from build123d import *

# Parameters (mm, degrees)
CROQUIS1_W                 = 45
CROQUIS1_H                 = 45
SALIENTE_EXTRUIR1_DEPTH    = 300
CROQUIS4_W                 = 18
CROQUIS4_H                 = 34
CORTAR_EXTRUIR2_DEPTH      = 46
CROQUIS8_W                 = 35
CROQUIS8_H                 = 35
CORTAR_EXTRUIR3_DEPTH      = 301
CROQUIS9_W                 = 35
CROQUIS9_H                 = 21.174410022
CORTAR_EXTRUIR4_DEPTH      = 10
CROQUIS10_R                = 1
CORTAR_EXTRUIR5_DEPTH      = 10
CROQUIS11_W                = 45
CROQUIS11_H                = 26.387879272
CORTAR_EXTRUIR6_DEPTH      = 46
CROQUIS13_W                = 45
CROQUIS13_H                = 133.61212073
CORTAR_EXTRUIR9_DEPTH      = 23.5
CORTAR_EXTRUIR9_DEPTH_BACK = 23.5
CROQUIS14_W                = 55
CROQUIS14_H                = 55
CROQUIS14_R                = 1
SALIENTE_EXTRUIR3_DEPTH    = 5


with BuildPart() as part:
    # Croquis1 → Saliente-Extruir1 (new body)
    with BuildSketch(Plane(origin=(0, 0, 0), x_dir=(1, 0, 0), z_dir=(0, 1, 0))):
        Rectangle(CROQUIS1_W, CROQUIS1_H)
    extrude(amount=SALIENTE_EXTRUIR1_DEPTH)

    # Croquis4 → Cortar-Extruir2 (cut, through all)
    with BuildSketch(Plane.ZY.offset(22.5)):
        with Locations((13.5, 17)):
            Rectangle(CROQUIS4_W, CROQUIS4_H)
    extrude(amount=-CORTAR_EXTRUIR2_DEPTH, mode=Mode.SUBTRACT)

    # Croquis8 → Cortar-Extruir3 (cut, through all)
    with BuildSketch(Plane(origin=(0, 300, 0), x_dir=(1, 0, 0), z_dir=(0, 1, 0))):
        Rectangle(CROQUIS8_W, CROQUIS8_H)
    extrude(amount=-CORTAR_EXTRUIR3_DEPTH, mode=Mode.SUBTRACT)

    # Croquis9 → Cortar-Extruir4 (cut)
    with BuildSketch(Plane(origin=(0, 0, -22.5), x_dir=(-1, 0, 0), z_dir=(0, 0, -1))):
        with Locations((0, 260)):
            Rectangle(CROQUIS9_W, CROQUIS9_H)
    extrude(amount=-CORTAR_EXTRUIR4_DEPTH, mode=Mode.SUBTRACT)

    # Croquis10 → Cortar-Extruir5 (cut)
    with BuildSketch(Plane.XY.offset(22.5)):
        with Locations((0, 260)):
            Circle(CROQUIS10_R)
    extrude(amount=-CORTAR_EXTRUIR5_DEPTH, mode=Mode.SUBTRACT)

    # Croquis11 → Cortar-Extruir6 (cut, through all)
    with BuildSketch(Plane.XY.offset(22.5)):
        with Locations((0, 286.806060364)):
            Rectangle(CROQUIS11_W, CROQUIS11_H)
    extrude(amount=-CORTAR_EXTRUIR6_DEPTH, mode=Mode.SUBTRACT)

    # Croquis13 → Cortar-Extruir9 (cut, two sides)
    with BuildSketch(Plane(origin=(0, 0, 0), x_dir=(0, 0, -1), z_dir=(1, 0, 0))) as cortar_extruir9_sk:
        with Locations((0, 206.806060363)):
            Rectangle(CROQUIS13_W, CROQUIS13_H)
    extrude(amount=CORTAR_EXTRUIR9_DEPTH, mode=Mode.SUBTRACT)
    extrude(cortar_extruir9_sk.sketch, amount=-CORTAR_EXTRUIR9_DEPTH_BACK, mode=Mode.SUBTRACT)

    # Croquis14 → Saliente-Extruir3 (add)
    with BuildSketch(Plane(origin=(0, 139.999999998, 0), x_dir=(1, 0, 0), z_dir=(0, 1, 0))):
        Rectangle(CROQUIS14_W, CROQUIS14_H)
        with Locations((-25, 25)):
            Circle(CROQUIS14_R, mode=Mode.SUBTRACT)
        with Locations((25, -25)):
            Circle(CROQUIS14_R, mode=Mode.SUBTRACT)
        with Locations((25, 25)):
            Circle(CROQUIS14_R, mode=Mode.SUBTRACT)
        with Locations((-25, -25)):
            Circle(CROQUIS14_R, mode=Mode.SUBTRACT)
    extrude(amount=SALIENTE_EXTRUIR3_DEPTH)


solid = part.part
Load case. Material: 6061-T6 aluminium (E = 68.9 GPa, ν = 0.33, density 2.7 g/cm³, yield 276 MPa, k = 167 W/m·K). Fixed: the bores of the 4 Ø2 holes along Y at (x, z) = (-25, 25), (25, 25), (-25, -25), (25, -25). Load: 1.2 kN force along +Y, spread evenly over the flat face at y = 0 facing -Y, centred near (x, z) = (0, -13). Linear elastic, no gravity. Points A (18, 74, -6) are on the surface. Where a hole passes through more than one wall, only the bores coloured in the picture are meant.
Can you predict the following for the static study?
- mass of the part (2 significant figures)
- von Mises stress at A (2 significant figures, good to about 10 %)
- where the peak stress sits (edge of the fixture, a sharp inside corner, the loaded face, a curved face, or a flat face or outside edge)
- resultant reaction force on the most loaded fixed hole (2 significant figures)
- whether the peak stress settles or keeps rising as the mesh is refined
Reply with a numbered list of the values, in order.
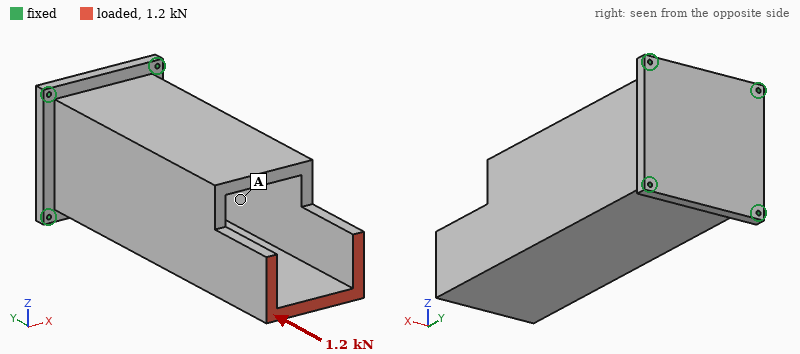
1. 310 g
2. 2.0 MPa
3. edge of the fixture
4. 490 N
5. keeps rising
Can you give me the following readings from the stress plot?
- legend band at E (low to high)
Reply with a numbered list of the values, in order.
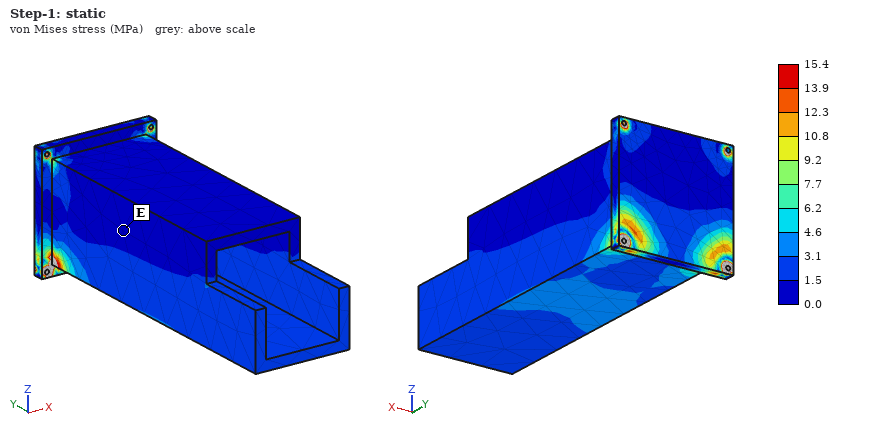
1. 0.0 to 1.5 MPa
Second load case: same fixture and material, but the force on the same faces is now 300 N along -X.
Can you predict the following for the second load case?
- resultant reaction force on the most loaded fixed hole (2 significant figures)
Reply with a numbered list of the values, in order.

1. 480 N
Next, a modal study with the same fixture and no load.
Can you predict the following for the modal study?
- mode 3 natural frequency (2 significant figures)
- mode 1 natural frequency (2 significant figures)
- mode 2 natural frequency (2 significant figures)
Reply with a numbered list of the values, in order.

1. 3900 Hz
2. 1300 Hz
3. 1300 Hz
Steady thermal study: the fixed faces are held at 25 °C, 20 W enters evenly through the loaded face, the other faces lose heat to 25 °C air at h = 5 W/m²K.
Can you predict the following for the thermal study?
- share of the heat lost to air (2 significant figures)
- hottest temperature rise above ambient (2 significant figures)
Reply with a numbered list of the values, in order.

1. 14 %
2. 30 K
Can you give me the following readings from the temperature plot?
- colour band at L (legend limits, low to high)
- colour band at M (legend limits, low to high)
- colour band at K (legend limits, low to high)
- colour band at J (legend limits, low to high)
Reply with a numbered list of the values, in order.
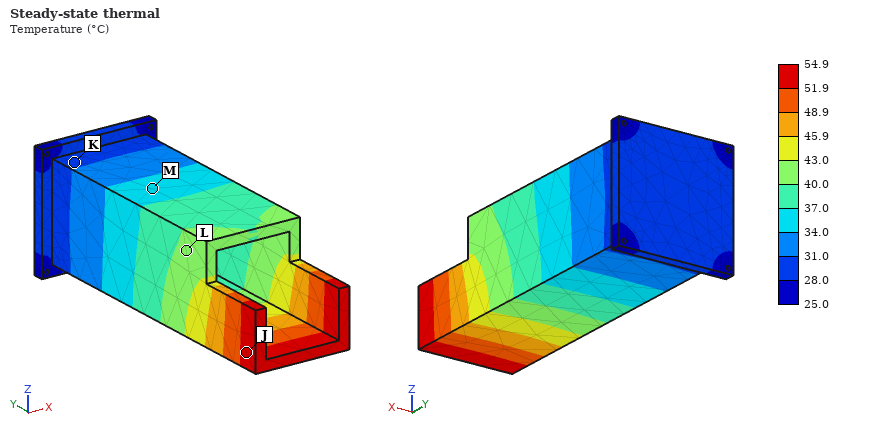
1. 40.0 to 43.0 °C
2. 34.0 to 37.0 °C
3. 28.0 to 31.0 °C
4. 51.9 to 54.9 °C
